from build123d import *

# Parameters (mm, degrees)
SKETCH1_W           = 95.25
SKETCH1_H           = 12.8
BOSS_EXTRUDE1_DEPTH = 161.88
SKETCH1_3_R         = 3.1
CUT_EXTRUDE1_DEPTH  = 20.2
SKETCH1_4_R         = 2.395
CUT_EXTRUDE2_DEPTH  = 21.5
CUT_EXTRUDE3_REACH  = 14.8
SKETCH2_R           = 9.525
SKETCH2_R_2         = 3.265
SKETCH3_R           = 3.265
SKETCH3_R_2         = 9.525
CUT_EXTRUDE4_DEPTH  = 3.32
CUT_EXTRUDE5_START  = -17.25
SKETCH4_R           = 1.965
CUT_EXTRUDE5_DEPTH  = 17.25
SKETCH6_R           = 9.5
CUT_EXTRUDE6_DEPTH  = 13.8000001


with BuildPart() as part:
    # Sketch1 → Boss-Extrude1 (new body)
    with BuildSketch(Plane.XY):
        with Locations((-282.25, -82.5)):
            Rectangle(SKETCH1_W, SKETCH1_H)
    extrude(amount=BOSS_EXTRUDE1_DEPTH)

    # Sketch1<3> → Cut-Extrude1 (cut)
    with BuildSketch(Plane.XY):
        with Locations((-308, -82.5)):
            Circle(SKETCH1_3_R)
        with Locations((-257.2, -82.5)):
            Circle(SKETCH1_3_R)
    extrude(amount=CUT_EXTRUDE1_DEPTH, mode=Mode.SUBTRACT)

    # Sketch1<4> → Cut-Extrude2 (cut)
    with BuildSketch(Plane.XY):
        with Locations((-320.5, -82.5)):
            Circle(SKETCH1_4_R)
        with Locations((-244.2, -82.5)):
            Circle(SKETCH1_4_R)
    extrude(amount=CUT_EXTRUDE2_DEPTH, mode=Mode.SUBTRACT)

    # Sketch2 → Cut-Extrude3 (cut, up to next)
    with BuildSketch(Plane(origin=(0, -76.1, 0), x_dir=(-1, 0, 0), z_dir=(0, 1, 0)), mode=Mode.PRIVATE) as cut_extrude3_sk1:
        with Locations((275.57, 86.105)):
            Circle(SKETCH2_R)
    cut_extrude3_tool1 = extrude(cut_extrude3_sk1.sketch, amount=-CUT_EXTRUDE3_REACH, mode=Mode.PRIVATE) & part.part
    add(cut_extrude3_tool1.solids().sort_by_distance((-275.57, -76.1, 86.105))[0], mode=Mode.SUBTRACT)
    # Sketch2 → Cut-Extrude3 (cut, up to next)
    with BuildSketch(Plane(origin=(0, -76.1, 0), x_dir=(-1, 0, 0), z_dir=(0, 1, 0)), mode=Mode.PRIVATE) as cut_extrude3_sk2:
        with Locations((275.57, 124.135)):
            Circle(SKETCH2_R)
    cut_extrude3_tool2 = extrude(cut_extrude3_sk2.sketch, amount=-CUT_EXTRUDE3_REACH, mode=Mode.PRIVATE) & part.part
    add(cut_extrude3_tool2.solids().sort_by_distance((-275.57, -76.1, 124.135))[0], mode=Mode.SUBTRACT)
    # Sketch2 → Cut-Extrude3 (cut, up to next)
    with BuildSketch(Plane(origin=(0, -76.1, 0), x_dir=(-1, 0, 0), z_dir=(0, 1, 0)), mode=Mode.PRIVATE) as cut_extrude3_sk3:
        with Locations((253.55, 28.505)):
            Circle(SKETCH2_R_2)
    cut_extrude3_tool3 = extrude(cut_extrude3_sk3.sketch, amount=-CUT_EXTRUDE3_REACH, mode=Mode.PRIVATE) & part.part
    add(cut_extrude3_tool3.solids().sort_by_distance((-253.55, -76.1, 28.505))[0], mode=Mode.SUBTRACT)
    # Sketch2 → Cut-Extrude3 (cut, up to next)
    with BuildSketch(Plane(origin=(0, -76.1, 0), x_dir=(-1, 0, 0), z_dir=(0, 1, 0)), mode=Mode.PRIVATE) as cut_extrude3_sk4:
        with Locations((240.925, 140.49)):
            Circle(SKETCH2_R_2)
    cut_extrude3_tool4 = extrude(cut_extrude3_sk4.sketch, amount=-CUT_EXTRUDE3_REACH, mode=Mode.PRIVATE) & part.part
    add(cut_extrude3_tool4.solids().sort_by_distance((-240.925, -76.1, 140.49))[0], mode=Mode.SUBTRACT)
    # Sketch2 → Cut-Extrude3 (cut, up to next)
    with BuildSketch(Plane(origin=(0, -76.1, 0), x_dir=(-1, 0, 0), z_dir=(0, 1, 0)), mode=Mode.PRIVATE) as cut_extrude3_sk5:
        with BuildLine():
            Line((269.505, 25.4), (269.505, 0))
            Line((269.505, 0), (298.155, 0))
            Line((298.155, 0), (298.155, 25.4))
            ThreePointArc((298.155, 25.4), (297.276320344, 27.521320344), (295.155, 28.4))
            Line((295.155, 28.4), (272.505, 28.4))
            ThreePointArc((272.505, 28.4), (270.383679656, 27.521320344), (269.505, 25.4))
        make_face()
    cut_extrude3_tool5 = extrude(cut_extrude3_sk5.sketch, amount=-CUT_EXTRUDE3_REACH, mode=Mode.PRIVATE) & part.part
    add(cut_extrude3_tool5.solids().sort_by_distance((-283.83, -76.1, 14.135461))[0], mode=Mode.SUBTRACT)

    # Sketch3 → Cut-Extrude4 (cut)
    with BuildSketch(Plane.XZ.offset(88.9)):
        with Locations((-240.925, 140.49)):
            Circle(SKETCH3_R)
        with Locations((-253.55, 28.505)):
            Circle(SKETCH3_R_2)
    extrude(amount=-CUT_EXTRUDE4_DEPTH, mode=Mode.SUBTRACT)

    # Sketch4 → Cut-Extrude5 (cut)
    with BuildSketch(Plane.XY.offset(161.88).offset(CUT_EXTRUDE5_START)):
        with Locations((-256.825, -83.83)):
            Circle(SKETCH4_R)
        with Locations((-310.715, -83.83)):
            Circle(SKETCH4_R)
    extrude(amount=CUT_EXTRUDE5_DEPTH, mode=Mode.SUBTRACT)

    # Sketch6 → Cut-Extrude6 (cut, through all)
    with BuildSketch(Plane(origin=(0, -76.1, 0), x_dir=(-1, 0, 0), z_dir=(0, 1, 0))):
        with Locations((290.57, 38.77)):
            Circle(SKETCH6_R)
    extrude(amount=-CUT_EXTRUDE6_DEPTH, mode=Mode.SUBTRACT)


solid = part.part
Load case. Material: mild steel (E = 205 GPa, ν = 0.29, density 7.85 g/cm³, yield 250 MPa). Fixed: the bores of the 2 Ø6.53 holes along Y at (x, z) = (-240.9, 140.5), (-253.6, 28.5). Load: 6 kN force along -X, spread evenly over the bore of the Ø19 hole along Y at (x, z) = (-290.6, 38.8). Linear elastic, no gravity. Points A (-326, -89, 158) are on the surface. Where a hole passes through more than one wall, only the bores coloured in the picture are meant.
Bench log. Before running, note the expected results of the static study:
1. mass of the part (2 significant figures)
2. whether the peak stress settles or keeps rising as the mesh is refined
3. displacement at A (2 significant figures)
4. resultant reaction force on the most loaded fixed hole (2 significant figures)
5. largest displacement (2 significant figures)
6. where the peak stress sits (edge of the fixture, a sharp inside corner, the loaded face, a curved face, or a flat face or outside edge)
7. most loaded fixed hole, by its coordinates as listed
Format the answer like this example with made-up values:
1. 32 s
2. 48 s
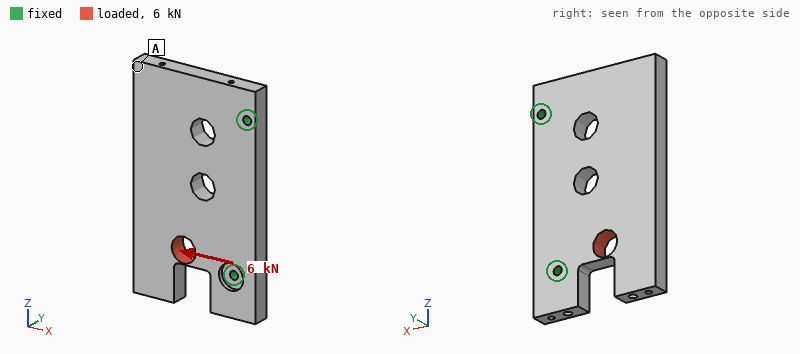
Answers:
1. 1.3 kg
2. keeps rising
3. 4.1 µm
4. 5.5 kN
5. 15 µm
6. a sharp inside corner
7. (-253.6, 28.5)
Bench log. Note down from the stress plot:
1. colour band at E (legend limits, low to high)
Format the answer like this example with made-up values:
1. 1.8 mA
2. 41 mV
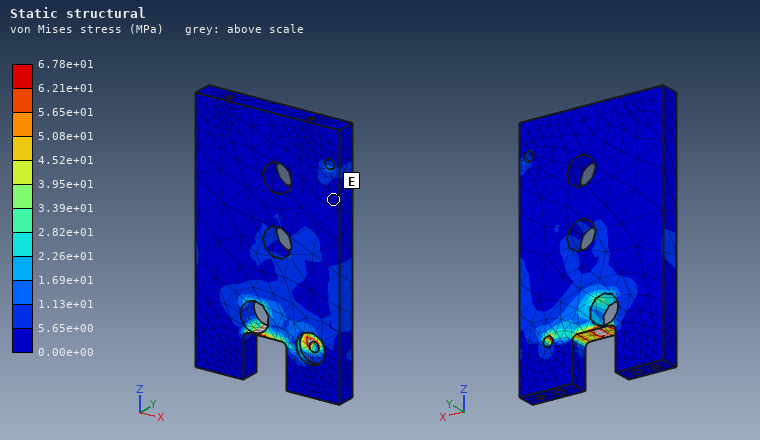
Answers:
1. 0.00e+00 to 5.65e+00 MPa
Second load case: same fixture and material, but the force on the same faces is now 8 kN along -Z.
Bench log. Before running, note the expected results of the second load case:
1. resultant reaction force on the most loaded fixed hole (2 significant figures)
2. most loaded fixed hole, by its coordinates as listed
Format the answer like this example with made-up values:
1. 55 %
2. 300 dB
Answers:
1. 5.9 kN
2. (-253.6, 28.5)
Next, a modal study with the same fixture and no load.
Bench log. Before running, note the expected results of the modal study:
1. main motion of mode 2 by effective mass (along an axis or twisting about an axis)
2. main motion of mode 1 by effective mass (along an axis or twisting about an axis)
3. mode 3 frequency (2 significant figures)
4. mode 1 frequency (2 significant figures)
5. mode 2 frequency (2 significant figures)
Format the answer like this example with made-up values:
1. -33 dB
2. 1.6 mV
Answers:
1. twisting about X
2. along Y
3. 3300 Hz
4. 910 Hz
5. 1700 Hz
